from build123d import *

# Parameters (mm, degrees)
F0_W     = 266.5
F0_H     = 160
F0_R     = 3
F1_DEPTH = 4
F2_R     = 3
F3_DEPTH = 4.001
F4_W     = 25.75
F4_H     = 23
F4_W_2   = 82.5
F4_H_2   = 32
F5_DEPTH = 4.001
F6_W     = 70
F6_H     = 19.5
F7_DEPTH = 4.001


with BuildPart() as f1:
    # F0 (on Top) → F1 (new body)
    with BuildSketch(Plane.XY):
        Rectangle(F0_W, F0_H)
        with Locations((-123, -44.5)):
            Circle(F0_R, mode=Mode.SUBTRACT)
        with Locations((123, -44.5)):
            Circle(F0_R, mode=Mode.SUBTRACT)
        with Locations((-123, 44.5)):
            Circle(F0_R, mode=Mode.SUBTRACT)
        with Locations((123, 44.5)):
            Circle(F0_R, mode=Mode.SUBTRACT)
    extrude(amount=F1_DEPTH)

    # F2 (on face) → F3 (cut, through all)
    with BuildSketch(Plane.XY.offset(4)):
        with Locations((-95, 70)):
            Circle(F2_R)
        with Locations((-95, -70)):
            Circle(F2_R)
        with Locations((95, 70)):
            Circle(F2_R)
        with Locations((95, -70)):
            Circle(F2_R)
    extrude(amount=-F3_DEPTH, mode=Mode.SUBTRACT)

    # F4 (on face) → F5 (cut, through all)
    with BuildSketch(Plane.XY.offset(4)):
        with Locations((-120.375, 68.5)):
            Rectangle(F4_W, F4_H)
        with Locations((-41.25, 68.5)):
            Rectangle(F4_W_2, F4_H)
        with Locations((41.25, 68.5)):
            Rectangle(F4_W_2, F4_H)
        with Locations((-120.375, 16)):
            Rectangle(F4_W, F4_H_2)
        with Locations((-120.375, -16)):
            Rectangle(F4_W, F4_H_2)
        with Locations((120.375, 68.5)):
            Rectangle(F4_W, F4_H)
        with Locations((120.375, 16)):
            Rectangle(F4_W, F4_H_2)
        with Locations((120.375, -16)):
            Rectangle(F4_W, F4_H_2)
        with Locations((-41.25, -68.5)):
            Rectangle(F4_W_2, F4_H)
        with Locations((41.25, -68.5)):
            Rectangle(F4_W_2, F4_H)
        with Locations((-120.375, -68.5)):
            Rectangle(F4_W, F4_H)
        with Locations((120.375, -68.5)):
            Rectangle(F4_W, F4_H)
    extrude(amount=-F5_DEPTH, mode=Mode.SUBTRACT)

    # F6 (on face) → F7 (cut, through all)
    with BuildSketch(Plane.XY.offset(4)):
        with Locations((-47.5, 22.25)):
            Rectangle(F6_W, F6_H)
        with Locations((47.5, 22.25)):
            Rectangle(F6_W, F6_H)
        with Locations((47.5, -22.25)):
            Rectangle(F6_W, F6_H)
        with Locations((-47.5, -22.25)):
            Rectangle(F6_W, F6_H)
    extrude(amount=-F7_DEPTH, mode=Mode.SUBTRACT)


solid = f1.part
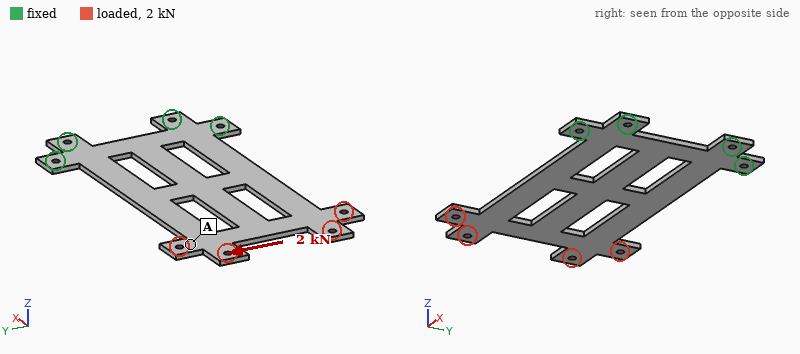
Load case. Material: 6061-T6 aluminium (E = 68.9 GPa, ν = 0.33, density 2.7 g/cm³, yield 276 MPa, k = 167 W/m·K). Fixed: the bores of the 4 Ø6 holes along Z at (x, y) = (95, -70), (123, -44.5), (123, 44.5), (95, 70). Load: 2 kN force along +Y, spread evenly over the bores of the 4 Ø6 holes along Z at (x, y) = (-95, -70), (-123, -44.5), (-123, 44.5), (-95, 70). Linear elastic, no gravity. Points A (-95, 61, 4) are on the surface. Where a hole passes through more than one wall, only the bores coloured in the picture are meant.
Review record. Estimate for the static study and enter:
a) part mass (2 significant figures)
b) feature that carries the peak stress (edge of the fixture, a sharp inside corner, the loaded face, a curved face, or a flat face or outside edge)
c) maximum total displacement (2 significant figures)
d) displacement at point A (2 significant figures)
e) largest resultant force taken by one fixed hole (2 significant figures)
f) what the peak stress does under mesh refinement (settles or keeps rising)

260 g
a sharp inside corner
0.59 mm
0.50 mm
2.3 kN
keeps rising
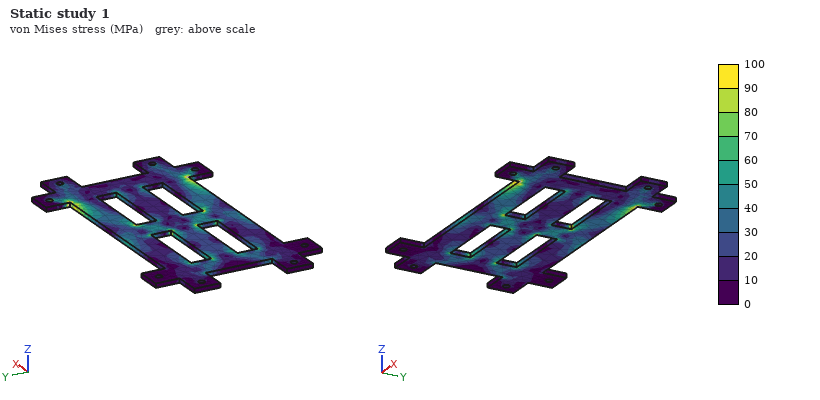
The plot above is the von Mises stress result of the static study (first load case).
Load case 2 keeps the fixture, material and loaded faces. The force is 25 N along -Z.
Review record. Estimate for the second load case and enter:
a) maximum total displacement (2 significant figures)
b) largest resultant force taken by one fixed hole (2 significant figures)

3.3 mm
59 N
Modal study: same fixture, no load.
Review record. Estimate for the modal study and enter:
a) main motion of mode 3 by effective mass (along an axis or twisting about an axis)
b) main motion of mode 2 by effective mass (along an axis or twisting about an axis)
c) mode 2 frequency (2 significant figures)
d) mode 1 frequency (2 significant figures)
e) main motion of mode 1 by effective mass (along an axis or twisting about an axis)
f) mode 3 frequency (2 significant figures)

along Z
twisting about X
200 Hz
54 Hz
along Z
350 Hz
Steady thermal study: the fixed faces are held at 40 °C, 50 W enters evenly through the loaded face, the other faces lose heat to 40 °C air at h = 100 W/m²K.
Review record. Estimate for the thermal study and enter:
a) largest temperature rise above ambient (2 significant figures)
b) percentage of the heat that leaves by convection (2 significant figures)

39 K
98 %
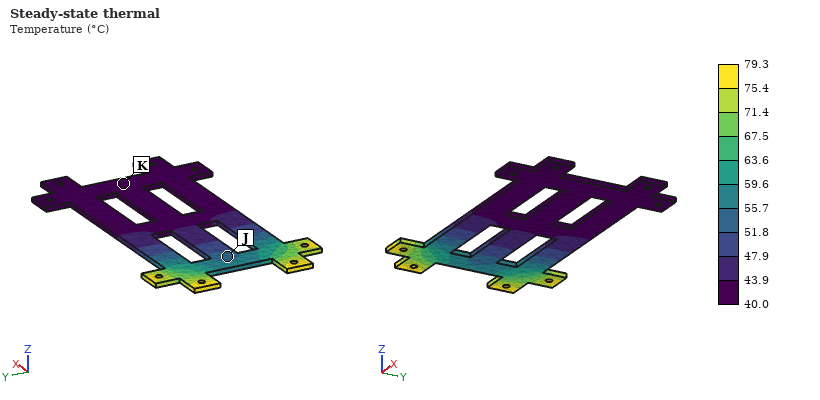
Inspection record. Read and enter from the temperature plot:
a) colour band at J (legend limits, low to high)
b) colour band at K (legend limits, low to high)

51.8 to 55.7 °C
40.0 to 43.9 °C
